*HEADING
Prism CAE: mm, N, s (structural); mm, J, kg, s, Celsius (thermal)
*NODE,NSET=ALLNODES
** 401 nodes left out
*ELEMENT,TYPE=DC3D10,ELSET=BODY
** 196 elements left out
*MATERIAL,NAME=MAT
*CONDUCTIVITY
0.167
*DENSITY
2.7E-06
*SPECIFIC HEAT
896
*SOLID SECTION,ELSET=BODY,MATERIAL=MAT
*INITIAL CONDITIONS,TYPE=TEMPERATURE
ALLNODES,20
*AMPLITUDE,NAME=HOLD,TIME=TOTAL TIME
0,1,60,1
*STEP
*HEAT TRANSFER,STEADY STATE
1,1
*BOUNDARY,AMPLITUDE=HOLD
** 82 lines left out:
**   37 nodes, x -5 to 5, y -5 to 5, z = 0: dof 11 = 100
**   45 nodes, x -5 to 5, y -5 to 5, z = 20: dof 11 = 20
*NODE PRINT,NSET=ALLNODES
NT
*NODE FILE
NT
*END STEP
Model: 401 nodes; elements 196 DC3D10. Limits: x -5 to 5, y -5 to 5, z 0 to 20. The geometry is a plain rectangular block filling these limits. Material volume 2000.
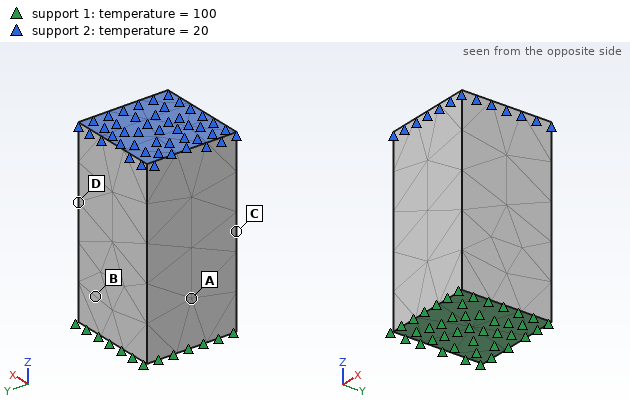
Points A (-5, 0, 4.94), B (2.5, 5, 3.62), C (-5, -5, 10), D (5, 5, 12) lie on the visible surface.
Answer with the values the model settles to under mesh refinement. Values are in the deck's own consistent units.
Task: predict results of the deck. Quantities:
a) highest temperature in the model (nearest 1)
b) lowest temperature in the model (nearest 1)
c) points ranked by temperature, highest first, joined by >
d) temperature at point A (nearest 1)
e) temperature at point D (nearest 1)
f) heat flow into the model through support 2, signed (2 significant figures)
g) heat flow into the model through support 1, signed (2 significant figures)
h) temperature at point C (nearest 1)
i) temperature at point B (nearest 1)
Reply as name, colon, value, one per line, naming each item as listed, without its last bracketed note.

highest temperature in the model: 100
lowest temperature in the model: 20
points ranked by temperature, highest first, joined by >: B > A > C > D
temperature at point A: 80
temperature at point D: 52
heat flow into the model through support 2, signed: -67
heat flow into the model through support 1, signed: 67
temperature at point C: 60
temperature at point B: 86
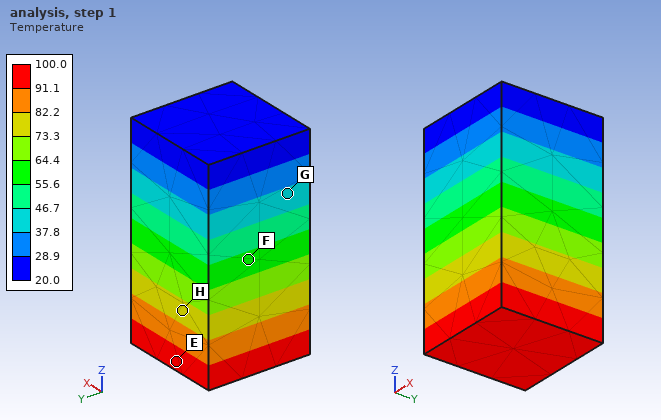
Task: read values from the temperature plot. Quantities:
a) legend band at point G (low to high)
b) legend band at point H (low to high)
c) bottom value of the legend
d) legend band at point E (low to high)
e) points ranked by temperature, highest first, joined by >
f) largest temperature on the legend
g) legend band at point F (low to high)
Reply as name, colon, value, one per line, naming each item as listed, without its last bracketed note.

legend band at point G: 37.8 to 46.7
legend band at point H: 73.3 to 82.2
bottom value of the legend: 20.0
legend band at point E: 91.1 to 100.0
points ranked by temperature, highest first, joined by >: E > H > F > G
largest temperature on the legend: 100.0
legend band at point F: 55.6 to 64.4
